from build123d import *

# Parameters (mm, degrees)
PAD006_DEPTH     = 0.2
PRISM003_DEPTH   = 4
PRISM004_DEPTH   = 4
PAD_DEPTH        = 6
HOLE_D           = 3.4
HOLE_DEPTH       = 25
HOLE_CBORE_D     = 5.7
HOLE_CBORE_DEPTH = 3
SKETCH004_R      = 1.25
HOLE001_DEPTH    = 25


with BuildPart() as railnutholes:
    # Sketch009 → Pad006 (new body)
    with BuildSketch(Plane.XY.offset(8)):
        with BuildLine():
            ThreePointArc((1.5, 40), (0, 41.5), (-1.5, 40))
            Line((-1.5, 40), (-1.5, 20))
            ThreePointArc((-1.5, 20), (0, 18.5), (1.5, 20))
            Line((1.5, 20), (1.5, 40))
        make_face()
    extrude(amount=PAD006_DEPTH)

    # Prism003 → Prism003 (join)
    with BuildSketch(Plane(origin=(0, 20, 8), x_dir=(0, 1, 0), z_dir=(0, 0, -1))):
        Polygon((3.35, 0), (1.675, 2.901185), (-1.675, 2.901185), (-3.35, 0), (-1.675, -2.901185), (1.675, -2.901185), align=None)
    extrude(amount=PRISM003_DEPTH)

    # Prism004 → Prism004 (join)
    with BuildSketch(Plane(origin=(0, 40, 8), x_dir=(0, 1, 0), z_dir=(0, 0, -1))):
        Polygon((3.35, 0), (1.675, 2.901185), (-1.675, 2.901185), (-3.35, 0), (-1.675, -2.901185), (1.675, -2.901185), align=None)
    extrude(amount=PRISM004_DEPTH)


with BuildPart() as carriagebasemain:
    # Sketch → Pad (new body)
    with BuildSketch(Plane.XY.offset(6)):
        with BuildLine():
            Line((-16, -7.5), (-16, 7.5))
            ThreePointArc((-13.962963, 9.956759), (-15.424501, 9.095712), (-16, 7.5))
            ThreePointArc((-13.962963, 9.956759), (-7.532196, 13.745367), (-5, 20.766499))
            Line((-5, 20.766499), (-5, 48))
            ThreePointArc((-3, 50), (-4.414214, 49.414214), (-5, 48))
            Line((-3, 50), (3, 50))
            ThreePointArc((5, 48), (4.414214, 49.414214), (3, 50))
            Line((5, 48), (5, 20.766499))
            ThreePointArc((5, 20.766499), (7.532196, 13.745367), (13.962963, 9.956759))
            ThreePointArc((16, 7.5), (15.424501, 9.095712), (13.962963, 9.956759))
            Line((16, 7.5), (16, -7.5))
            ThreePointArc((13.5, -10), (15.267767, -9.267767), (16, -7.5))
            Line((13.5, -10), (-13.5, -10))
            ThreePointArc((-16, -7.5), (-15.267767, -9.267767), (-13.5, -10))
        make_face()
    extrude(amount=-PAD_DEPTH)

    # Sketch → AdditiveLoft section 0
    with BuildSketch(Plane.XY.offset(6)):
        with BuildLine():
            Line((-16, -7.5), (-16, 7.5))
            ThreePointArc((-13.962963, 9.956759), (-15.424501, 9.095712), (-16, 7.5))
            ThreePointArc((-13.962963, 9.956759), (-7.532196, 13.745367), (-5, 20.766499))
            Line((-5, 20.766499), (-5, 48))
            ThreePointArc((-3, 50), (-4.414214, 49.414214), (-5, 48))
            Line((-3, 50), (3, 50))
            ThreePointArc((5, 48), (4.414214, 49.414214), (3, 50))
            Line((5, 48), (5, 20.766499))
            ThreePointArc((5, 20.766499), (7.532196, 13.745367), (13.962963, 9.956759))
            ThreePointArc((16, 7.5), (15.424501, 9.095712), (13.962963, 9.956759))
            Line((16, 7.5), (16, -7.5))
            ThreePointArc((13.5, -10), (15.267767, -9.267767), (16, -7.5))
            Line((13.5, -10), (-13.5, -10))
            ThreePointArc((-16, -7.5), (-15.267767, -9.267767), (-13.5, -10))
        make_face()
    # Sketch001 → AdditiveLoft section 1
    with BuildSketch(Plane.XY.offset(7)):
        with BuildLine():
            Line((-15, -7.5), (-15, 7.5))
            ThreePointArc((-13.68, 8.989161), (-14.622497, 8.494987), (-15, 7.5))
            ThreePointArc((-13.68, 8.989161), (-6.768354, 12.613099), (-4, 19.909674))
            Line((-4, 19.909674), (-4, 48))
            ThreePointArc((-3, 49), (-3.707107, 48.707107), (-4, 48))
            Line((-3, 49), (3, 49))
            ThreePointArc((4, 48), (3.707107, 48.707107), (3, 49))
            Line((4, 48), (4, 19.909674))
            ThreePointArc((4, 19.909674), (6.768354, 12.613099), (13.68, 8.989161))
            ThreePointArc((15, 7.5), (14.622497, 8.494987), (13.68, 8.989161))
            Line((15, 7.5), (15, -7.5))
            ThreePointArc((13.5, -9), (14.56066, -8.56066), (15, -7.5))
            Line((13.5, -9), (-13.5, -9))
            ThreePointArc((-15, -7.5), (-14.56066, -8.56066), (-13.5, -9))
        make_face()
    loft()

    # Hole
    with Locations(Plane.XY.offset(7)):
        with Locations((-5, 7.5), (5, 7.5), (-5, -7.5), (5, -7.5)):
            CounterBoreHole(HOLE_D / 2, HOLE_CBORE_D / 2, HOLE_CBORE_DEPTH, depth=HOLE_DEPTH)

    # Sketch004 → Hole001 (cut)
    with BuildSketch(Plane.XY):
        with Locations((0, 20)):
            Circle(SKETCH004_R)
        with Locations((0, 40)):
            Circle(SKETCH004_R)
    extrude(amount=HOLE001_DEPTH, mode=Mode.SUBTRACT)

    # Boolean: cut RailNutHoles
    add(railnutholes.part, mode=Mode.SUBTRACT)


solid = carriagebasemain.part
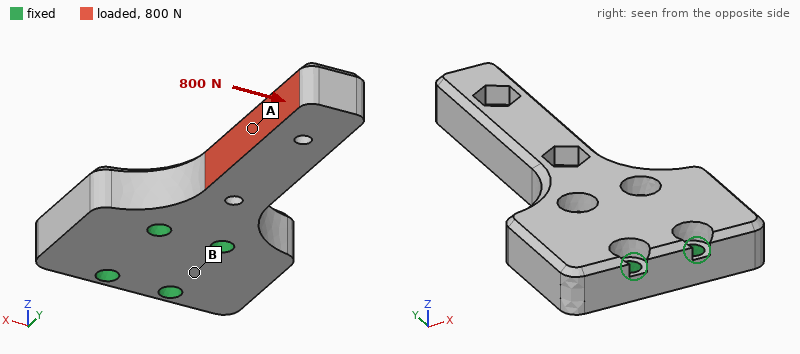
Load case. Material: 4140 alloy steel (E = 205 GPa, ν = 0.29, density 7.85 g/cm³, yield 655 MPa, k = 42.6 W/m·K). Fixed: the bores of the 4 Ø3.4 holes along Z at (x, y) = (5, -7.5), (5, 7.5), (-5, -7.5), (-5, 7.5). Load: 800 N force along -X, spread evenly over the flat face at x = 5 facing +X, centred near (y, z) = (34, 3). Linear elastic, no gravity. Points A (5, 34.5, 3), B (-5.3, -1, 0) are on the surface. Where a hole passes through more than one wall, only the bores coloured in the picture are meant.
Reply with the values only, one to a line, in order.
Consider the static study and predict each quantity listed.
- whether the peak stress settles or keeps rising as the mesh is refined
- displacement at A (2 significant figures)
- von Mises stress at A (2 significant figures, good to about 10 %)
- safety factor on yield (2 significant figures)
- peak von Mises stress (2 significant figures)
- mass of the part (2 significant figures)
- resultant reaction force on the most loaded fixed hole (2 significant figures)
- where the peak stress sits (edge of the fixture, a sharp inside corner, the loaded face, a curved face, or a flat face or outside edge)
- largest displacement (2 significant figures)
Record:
settles
28 µm
29 MPa
4.4
150 MPa
54 g
1.4 kN
a curved face
55 µm
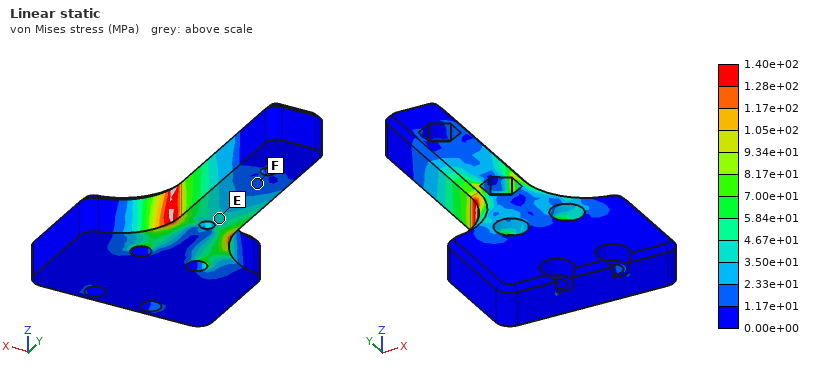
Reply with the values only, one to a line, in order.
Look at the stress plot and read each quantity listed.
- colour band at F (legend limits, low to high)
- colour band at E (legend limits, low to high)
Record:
1.17e+01 to 2.33e+01 MPa
3.50e+01 to 4.67e+01 MPa
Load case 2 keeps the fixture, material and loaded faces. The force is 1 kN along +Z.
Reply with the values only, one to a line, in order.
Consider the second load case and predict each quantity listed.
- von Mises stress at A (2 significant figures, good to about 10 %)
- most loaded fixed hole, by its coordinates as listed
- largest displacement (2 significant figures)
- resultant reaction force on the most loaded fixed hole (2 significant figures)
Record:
55 MPa
(5, 7.5)
0.26 mm
1.6 kN
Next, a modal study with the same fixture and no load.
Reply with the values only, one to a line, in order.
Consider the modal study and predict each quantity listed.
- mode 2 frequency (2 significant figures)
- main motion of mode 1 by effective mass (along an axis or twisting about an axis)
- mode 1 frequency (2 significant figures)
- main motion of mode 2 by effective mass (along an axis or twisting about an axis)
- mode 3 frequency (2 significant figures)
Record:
5900 Hz
along Z
3100 Hz
along X
17 kHz
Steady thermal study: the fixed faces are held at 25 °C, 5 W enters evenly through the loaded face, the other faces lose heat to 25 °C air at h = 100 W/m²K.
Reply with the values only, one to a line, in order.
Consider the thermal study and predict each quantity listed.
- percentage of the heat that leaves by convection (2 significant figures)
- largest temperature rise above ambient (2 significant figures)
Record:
47 %
27 K
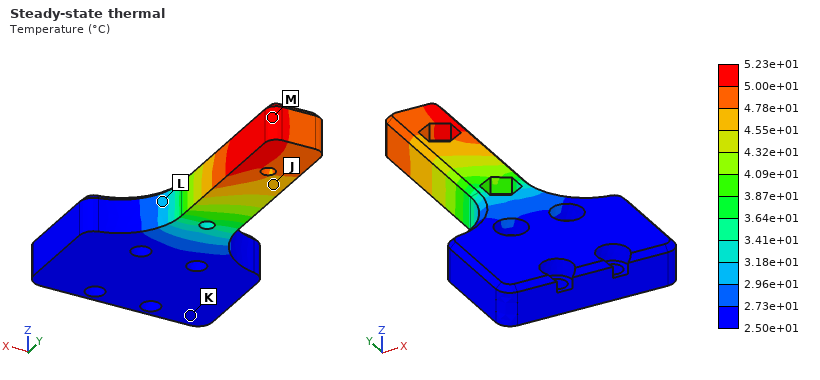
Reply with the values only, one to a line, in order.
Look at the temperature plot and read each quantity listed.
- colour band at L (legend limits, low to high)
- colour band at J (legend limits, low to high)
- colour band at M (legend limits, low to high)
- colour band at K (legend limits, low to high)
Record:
2.96e+01 to 3.18e+01 °C
4.55e+01 to 4.78e+01 °C
5.00e+01 to 5.23e+01 °C
2.50e+01 to 2.73e+01 °C
